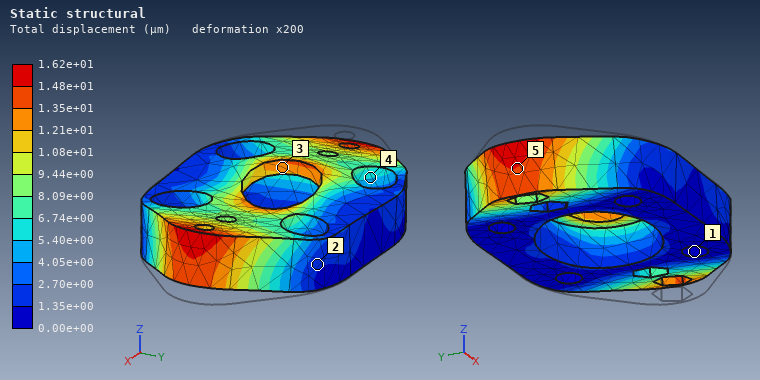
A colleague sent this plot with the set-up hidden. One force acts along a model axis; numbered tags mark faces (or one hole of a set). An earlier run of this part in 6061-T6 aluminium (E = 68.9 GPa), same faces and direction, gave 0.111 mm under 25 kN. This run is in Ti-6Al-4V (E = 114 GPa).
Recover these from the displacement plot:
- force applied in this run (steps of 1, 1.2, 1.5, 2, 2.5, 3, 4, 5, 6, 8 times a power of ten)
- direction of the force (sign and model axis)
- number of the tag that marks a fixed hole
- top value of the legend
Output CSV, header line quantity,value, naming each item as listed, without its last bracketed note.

quantity,value
force applied in this run,6 kN
direction of the force,-X
number of the tag that marks a fixed hole,1
top value of the legend,1.62e+01 µm
